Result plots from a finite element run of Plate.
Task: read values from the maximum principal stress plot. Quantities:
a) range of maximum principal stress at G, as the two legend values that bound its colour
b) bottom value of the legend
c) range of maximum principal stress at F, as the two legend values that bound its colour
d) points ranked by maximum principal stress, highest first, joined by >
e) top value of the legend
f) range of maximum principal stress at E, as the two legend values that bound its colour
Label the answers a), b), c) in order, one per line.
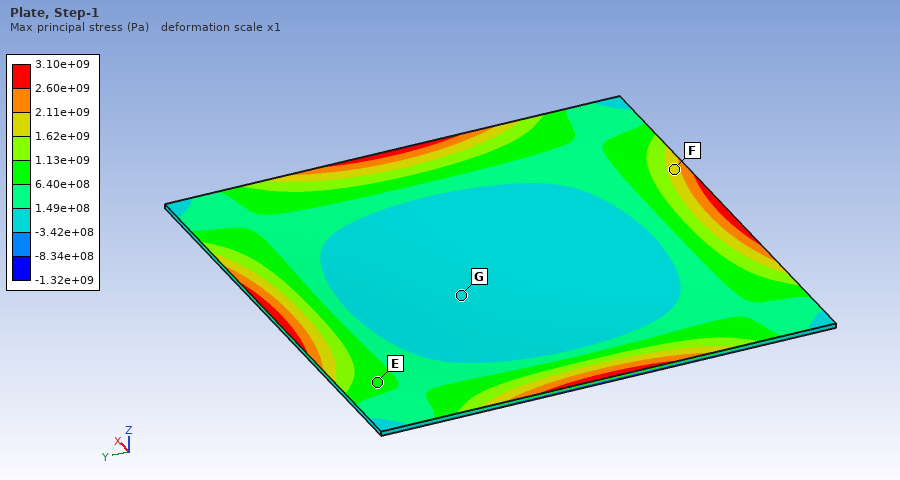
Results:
a) -3.42e+08 to 1.49e+08 Pa
b) -1.32e+09 Pa
c) 1.62e+09 to 2.11e+09 Pa
d) F > E > G
e) 3.10e+09 Pa
f) 6.40e+08 to 1.13e+09 Pa
